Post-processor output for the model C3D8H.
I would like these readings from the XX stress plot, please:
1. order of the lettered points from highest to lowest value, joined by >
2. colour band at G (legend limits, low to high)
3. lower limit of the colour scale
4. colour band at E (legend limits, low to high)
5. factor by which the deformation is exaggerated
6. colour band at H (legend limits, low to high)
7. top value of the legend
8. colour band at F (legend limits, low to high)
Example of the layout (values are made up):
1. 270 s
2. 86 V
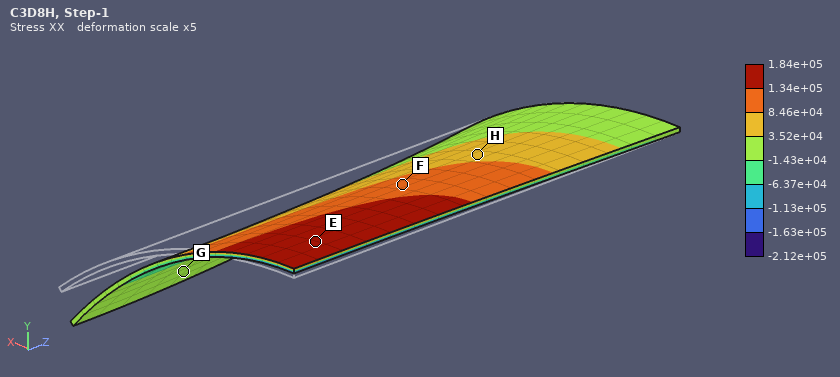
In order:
1. E > F > H > G
2. -1.43e+04 to 3.52e+04
3. -2.12e+05
4. 1.34e+05 to 1.84e+05
5. 5
6. 3.52e+04 to 8.46e+04
7. 1.84e+05
8. 8.46e+04 to 1.34e+05
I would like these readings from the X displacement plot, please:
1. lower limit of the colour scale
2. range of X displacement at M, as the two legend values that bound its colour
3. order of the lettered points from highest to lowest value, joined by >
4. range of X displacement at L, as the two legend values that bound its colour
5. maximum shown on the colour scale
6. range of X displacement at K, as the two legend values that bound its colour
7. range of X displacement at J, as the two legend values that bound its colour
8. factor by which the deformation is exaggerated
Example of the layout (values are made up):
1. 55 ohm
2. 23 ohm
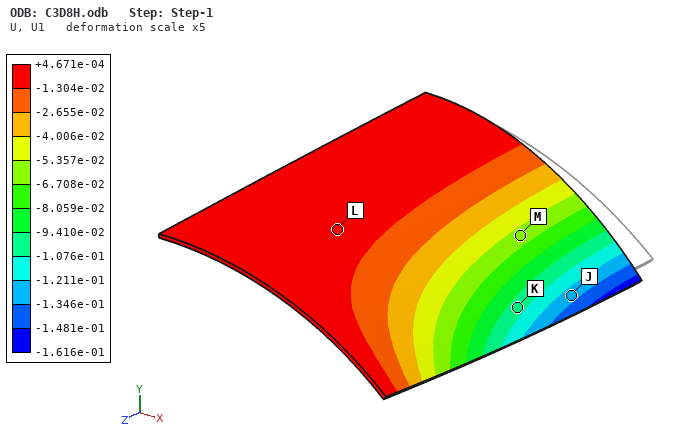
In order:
1. -1.616e-01
2. -6.708e-02 to -5.357e-02
3. L > M > K > J
4. -1.304e-02 to +4.671e-04
5. +4.671e-04
6. -1.076e-01 to -9.410e-02
7. -1.346e-01 to -1.211e-01
8. 5
